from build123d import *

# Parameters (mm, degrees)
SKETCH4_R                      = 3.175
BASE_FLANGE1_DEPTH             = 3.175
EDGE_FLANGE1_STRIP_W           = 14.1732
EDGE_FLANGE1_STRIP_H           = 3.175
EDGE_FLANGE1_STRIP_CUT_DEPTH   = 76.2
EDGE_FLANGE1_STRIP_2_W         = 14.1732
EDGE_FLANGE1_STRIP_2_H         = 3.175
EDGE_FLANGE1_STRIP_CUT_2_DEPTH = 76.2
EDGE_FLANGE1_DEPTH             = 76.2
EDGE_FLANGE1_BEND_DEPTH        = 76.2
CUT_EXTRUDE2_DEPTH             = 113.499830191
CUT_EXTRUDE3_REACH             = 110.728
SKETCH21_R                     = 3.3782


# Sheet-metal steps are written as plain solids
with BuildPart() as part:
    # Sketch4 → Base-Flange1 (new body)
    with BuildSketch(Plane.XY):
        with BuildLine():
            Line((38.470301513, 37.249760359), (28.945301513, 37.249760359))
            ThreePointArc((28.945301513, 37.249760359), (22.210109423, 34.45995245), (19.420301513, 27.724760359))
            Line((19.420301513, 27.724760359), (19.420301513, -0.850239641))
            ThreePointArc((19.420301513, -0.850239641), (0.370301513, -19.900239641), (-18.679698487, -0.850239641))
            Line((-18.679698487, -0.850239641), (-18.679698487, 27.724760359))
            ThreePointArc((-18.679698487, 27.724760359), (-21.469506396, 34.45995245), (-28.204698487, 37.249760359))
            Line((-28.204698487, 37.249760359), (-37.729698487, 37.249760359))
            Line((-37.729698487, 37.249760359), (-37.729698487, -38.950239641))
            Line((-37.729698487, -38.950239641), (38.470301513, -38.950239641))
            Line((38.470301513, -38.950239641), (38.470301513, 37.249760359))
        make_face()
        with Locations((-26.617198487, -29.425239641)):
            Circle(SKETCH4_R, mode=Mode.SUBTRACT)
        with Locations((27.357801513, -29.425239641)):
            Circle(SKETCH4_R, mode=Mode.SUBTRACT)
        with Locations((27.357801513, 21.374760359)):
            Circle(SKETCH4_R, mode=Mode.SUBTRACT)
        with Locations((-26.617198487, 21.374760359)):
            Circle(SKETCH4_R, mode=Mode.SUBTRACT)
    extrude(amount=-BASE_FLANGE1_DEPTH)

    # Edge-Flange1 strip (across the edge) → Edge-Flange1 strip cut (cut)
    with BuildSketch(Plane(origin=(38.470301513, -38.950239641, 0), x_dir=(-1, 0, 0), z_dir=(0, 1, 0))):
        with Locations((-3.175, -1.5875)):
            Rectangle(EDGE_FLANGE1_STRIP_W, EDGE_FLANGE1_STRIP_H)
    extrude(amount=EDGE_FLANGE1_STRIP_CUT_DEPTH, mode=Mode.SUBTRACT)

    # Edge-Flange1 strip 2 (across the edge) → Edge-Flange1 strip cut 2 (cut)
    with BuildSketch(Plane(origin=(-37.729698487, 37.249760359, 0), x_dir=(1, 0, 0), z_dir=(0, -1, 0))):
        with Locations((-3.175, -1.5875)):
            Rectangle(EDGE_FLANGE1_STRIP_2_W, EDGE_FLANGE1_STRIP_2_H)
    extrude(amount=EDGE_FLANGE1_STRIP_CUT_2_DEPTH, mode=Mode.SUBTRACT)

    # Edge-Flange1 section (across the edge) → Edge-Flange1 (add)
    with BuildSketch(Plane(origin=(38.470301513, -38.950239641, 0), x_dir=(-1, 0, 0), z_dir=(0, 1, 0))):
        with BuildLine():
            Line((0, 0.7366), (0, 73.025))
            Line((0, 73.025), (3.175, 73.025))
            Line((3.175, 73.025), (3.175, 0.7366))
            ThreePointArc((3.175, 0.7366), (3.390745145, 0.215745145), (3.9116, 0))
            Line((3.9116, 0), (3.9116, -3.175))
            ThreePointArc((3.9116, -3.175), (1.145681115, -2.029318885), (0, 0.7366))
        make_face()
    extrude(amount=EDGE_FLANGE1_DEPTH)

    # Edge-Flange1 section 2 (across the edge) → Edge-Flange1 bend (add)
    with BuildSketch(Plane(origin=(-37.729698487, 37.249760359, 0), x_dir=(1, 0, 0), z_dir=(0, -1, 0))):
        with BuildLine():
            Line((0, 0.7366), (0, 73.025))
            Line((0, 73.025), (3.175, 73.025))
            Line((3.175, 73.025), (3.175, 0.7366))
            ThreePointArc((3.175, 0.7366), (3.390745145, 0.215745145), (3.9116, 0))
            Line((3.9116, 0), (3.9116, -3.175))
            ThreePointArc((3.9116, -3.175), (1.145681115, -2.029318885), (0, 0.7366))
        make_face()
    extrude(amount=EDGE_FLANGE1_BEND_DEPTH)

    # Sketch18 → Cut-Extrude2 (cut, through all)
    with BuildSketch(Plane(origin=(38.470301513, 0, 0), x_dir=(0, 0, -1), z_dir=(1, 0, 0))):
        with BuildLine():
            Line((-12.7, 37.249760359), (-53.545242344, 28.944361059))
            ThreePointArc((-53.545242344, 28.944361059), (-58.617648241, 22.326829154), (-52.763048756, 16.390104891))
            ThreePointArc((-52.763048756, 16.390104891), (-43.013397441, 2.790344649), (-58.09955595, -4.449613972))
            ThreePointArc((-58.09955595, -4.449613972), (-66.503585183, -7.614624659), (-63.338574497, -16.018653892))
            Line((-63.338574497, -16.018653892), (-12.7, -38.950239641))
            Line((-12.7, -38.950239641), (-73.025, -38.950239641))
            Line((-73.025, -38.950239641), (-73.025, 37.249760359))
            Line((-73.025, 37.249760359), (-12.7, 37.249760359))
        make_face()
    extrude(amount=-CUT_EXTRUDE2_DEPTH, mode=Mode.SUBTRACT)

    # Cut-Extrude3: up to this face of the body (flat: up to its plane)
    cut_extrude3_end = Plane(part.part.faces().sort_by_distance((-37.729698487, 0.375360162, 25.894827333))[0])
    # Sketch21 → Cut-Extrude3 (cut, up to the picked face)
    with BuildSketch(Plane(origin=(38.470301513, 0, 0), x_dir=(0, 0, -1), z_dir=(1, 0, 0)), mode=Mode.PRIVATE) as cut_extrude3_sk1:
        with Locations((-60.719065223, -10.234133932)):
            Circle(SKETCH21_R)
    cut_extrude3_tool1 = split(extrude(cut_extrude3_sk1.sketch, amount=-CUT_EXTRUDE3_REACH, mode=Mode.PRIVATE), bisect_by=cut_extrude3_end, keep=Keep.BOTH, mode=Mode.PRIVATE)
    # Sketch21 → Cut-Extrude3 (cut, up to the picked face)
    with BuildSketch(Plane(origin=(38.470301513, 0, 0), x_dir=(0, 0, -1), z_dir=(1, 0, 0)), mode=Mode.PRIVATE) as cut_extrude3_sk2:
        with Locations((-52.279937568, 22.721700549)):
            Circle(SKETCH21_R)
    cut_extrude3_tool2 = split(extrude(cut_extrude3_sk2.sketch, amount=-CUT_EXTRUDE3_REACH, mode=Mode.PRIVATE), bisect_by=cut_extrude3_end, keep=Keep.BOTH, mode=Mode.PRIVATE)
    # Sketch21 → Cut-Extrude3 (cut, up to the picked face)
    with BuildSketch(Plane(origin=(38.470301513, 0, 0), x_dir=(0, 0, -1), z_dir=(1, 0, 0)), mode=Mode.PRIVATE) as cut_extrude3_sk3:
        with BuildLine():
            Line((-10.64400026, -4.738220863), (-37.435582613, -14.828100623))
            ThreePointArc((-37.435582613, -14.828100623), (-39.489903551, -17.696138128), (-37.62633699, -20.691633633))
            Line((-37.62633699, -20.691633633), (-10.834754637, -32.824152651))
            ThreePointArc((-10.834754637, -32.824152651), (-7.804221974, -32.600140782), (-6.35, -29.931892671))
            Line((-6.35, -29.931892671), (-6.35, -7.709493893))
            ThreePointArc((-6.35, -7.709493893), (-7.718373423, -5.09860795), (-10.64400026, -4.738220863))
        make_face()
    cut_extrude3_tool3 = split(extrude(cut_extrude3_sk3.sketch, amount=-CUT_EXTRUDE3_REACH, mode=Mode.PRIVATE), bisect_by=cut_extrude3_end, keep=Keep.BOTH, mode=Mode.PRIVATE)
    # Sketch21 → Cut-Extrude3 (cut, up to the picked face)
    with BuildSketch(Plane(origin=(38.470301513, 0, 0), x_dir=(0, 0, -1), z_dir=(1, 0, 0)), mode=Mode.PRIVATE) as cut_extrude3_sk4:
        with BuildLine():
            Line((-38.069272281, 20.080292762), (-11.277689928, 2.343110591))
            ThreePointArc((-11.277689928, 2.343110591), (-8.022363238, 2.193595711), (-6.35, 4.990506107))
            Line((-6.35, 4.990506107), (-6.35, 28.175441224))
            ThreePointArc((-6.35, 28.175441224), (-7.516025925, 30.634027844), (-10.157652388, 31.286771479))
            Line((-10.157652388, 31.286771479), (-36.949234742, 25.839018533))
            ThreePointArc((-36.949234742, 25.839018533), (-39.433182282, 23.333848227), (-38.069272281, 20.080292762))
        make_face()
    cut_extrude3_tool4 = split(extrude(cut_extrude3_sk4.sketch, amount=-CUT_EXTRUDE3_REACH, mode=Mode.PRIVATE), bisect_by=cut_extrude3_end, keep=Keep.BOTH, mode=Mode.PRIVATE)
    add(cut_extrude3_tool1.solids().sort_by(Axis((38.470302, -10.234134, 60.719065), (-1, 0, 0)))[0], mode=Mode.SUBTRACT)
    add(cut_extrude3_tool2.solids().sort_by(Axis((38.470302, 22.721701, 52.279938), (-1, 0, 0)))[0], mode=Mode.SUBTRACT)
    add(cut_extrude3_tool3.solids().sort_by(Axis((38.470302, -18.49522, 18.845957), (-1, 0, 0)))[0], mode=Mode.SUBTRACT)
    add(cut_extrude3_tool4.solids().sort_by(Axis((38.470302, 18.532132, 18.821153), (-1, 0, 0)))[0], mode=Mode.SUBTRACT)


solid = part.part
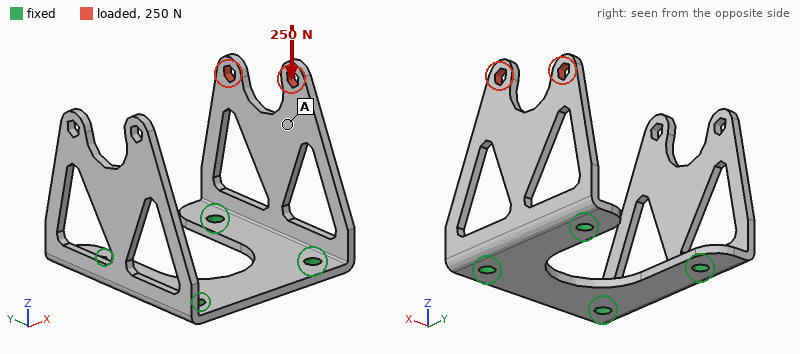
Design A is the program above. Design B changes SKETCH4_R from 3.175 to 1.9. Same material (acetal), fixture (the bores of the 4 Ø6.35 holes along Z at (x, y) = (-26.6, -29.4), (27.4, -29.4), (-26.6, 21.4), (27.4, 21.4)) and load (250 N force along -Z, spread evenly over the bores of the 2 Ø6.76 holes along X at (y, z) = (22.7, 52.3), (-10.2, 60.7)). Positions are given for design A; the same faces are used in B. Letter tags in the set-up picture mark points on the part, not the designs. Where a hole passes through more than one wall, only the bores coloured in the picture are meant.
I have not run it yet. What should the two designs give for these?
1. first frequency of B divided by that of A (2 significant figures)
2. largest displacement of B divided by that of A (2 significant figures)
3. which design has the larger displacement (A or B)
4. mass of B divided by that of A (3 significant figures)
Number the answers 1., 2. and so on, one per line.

1. 0.97
2. 1.4
3. B
4. 1.01
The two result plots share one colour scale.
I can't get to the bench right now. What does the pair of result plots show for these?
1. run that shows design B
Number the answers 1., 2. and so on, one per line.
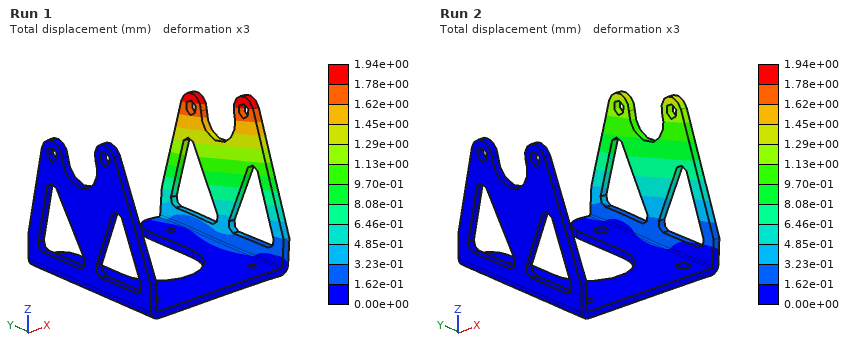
1. Run 1
